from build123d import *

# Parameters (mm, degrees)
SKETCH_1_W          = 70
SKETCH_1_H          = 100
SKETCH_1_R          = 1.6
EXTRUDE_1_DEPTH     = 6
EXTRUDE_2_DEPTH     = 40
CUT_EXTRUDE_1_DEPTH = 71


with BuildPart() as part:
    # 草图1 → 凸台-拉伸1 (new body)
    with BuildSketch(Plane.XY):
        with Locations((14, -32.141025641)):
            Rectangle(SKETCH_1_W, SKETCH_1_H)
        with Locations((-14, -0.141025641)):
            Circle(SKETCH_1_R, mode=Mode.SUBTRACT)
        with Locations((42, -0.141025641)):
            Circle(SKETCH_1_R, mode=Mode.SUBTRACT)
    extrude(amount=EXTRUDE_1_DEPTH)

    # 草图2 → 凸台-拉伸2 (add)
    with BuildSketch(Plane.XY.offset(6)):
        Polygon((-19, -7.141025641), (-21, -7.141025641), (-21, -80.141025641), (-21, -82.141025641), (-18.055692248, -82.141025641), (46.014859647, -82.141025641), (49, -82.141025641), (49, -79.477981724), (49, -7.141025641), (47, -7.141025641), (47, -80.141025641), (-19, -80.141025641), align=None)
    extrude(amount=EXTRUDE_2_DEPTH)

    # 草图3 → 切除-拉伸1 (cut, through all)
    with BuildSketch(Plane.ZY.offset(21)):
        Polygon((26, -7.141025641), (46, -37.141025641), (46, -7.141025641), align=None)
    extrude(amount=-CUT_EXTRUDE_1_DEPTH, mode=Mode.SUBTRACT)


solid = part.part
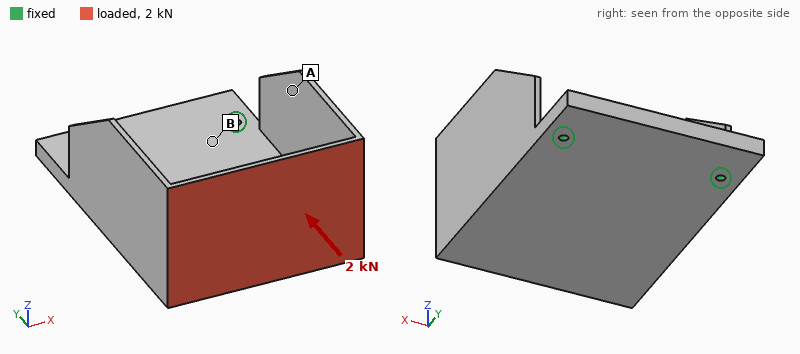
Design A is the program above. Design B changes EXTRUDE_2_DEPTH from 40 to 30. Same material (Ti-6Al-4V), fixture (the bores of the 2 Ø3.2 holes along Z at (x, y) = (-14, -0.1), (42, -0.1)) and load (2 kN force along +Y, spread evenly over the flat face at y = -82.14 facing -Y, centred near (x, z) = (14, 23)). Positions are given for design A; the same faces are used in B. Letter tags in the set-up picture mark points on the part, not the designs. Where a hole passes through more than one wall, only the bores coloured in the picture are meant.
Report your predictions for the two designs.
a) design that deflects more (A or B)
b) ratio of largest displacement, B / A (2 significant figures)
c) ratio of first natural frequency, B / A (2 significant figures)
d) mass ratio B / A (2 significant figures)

A
0.73
1.1
0.94
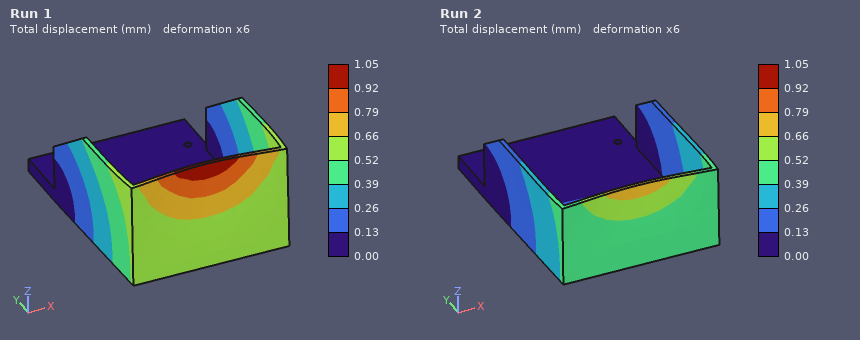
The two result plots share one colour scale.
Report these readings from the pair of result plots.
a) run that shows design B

Run 2
